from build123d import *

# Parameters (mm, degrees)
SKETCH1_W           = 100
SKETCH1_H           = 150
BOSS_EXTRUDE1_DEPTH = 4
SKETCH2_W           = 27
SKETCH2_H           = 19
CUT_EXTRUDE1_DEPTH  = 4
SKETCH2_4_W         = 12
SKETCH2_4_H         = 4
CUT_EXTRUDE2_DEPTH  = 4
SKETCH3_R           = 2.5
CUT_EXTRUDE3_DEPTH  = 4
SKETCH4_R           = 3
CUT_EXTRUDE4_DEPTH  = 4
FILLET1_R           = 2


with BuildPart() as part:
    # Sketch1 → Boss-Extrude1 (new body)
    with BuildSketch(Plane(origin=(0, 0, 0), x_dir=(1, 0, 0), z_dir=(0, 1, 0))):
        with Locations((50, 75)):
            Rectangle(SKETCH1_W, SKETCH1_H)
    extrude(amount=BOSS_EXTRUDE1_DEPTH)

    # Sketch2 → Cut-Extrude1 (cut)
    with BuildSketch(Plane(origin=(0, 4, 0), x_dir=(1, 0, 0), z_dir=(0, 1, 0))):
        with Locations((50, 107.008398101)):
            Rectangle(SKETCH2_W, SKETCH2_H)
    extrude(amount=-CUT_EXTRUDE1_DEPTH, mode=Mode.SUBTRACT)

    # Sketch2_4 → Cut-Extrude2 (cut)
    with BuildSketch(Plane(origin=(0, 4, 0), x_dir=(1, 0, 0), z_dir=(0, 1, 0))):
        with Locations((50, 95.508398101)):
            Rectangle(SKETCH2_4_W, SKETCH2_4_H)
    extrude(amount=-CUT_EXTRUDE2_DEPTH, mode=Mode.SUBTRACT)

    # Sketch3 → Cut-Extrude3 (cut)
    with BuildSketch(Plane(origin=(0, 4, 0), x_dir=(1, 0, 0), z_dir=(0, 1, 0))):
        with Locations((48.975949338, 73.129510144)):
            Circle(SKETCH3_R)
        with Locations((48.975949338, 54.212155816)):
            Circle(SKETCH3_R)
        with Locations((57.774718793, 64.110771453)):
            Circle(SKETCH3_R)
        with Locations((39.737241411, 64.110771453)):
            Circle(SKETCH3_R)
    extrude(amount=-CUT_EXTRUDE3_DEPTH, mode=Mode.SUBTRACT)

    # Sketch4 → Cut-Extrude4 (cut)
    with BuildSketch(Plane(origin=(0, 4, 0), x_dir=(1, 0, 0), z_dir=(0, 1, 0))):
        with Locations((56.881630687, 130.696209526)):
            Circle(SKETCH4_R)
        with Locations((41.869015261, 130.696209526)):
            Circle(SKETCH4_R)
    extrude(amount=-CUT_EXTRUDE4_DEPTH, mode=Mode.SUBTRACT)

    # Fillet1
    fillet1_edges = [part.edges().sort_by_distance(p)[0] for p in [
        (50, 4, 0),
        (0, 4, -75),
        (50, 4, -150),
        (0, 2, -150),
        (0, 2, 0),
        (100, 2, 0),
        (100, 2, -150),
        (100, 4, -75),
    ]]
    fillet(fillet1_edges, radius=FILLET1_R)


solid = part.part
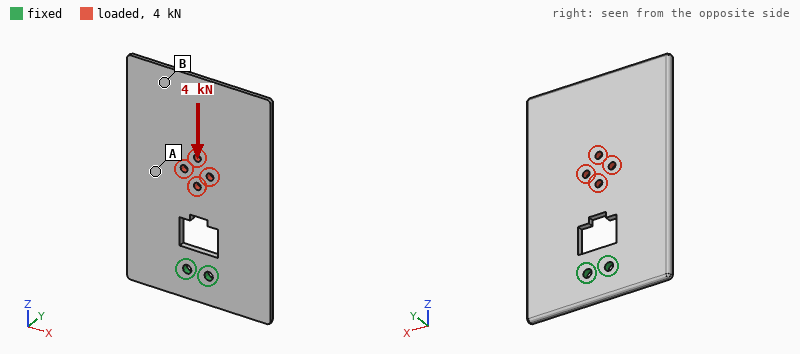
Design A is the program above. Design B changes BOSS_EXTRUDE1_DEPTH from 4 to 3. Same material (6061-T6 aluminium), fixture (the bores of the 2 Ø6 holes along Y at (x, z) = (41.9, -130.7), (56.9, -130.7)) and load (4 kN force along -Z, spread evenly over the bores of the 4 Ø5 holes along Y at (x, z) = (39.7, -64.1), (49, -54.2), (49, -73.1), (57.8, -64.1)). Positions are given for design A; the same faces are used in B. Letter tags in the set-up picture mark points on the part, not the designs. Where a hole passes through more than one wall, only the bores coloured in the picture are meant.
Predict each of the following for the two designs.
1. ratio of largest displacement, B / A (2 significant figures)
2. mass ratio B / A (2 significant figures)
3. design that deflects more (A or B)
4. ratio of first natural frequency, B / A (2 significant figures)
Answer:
1.3
0.75
B
0.76
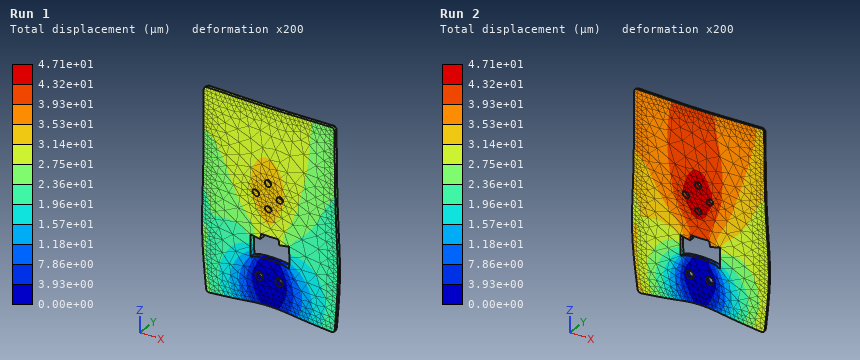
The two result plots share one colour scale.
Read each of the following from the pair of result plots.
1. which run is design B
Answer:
Run 2
